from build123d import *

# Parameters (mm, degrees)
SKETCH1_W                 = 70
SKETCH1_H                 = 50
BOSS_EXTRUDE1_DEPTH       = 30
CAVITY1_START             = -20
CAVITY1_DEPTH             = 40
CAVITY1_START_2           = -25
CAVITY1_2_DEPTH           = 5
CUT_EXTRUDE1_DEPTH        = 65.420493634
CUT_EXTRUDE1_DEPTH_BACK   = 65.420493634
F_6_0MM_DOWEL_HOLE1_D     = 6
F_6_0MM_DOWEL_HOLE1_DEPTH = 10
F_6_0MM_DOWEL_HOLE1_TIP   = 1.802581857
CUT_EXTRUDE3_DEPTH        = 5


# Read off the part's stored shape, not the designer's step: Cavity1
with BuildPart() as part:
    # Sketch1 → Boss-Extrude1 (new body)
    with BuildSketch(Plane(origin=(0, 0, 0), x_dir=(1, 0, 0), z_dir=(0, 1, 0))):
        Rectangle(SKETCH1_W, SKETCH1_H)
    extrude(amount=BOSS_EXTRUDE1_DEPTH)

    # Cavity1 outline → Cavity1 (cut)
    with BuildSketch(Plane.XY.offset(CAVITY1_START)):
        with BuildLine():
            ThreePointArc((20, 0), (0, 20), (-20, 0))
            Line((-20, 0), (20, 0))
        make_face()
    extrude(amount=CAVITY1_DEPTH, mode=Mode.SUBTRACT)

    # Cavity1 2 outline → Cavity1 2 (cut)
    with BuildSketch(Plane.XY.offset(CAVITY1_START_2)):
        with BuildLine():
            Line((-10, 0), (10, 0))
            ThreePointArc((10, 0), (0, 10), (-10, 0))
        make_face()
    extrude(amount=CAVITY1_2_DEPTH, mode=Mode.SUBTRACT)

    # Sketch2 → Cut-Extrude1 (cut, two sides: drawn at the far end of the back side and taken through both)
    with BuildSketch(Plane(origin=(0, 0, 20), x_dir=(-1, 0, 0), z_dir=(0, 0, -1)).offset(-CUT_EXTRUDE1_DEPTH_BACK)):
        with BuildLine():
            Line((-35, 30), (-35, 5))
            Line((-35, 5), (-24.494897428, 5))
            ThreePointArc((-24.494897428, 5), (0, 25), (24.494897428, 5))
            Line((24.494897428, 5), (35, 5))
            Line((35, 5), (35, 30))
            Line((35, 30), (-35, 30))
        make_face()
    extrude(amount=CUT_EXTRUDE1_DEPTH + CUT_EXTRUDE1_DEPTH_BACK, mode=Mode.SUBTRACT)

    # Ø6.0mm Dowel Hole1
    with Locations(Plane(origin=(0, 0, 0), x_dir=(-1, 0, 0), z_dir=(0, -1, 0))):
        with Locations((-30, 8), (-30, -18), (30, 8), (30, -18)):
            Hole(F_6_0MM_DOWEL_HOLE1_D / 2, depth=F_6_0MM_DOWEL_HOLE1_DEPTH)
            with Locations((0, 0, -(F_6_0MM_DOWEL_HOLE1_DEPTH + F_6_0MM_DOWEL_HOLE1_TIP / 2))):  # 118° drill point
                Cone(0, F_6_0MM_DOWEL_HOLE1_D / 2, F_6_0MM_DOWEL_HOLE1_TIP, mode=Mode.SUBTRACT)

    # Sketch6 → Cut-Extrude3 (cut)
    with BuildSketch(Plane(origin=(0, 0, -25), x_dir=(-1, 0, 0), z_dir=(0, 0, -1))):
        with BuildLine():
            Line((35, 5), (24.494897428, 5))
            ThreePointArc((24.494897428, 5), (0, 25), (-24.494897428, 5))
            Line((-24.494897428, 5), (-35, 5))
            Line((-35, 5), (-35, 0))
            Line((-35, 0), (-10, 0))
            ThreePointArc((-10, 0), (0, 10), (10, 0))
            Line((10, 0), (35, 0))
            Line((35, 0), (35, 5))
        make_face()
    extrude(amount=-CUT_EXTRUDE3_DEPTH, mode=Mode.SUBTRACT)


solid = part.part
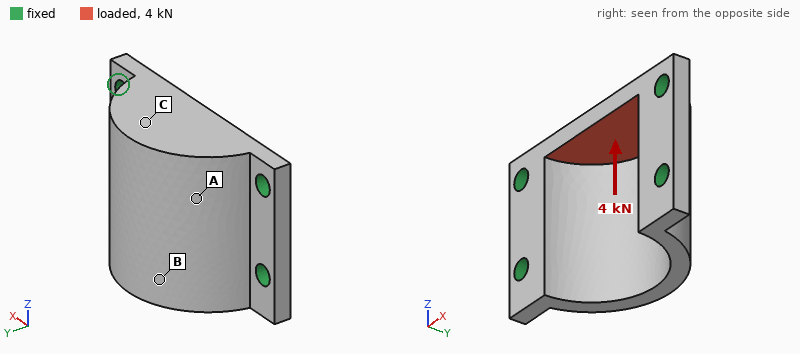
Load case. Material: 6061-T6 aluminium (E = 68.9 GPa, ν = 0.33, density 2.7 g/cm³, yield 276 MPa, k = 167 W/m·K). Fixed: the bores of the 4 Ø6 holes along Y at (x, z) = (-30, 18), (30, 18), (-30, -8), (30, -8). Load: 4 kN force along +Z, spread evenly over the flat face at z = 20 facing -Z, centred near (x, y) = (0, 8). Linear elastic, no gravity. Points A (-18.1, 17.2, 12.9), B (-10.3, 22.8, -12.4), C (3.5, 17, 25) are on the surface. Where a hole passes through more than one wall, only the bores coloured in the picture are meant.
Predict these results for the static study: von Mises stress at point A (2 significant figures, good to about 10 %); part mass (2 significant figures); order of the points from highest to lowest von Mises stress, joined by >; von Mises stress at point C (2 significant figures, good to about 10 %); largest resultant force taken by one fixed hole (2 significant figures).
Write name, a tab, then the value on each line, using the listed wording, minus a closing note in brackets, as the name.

von Mises stress at point A	20 MPa
part mass	62 g
order of the points from highest to lowest von Mises stress, joined by >	C > A > B
von Mises stress at point C	53 MPa
largest resultant force taken by one fixed hole	1.2 kN
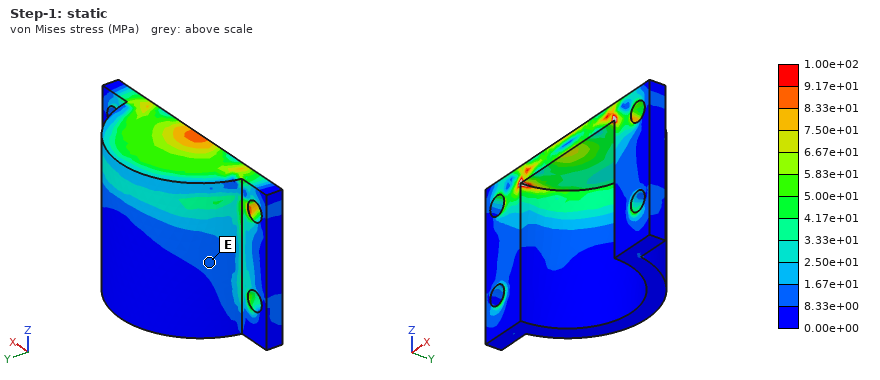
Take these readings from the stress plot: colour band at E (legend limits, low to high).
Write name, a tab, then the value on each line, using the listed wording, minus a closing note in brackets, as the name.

colour band at E	8.33e+00 to 1.67e+01 MPa
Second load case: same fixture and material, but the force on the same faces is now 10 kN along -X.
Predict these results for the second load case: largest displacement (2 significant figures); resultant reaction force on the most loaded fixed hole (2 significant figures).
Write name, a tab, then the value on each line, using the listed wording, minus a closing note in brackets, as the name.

largest displacement	39 µm
resultant reaction force on the most loaded fixed hole	4.6 kN
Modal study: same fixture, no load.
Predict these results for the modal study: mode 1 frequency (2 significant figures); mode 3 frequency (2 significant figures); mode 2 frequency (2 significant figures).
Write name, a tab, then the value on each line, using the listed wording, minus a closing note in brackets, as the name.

mode 1 frequency	10 kHz
mode 3 frequency	15 kHz
mode 2 frequency	10 kHz
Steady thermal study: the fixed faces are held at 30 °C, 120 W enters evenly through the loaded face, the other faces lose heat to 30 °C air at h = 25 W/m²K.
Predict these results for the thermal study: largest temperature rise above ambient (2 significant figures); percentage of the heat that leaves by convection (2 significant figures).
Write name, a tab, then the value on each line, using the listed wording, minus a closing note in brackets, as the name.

largest temperature rise above ambient	64 K
percentage of the heat that leaves by convection	4.0 %
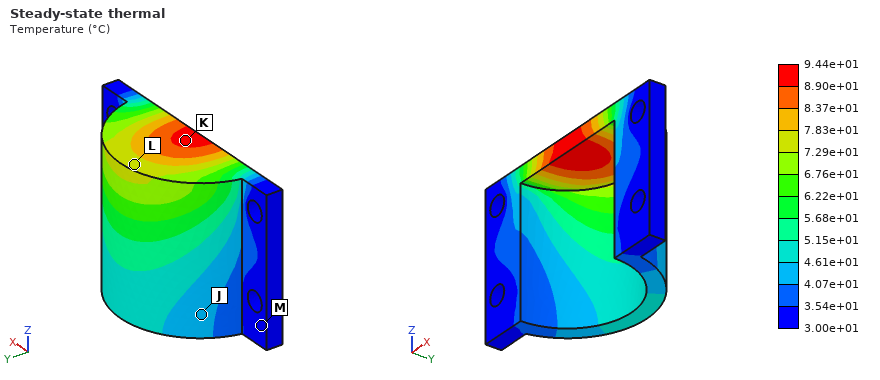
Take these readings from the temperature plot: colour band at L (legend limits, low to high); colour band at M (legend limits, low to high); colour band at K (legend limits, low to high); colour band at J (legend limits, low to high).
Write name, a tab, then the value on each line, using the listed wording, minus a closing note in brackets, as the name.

colour band at L	7.29e+01 to 7.83e+01 °C
colour band at M	3.00e+01 to 3.54e+01 °C
colour band at K	8.90e+01 to 9.44e+01 °C
colour band at J	4.07e+01 to 4.61e+01 °C
